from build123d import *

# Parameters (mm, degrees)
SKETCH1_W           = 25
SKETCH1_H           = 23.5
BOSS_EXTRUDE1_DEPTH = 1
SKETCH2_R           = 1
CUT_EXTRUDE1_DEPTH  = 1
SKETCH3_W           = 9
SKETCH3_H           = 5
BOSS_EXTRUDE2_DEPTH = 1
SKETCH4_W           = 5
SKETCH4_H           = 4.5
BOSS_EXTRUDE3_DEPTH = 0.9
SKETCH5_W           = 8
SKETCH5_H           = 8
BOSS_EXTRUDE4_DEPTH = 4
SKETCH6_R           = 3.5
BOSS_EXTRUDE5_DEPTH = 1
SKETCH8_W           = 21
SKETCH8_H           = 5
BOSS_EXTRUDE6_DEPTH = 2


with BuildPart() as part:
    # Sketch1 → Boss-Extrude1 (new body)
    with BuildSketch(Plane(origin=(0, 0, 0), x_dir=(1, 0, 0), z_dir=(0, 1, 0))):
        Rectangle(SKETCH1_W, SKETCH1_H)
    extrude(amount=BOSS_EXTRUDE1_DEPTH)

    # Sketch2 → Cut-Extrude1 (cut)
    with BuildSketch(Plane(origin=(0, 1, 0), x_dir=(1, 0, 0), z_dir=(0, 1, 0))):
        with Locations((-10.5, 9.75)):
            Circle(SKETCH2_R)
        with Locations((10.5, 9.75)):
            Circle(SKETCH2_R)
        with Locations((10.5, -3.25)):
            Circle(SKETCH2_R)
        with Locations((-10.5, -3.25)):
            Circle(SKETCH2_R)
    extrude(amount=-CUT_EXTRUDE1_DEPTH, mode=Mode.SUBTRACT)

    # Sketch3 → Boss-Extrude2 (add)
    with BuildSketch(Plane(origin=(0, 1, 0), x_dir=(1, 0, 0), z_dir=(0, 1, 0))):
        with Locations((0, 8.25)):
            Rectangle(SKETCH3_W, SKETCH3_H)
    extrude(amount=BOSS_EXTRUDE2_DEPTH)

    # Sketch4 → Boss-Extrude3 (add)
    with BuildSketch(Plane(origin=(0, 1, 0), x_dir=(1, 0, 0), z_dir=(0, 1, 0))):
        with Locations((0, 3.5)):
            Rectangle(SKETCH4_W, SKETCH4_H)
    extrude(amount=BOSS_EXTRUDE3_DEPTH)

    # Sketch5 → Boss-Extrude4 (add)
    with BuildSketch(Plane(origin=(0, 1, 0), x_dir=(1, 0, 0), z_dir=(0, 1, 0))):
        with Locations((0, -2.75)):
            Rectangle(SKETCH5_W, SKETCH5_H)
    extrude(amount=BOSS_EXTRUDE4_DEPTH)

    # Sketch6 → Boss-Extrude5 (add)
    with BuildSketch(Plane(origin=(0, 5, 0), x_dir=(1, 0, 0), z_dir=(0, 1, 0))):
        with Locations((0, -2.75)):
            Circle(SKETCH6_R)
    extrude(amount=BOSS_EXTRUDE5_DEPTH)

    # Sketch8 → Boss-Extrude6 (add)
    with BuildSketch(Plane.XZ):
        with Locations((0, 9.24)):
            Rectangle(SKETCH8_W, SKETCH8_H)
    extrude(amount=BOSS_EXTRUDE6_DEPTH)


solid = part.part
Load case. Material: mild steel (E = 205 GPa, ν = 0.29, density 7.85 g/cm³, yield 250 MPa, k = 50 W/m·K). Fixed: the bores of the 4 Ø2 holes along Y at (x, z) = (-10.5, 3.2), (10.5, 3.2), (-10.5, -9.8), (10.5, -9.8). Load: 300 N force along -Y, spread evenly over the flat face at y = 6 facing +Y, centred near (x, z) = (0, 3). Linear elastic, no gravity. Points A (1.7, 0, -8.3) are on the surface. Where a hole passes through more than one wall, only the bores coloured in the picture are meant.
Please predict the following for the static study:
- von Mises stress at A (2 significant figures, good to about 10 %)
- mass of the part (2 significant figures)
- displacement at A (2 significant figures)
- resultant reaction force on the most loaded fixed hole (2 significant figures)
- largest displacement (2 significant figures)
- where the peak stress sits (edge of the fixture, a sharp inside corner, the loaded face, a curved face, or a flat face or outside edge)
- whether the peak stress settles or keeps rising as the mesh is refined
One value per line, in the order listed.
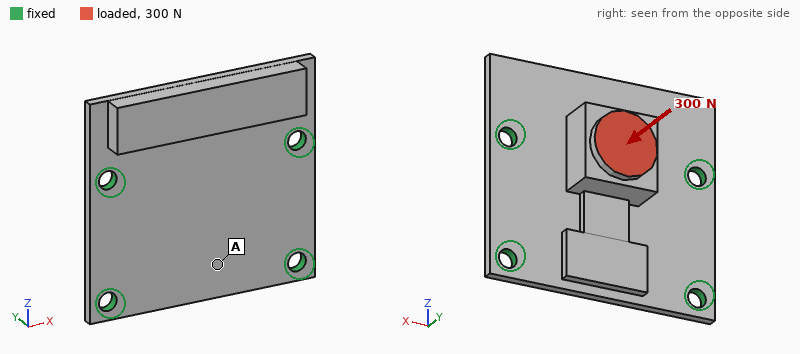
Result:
17 MPa
9.0 g
5.6 µm
140 N
15 µm
edge of the fixture
keeps rising
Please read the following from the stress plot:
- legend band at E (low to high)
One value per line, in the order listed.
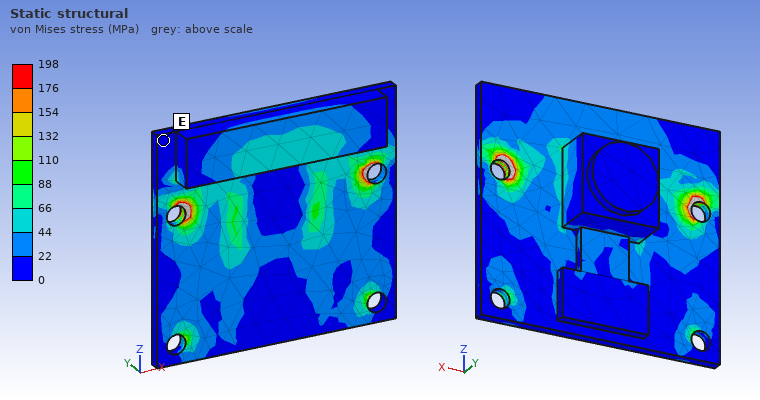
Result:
0 to 22 MPa
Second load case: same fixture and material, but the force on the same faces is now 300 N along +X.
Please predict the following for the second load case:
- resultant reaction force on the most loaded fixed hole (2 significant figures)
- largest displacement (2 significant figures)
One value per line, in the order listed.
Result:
140 N
7.6 µm
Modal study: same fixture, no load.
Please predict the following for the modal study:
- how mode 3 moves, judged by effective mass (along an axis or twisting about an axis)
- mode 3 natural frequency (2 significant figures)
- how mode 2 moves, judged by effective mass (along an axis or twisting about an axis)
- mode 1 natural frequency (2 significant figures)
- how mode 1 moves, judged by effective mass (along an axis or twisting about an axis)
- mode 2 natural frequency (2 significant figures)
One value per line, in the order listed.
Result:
twisting about Z
20 kHz
along Y
7800 Hz
along Y
12 kHz
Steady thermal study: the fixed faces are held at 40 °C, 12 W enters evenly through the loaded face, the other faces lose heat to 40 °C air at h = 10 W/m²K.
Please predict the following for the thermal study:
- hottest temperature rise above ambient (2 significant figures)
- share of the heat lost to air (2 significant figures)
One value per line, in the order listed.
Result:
79 K
3.9 %
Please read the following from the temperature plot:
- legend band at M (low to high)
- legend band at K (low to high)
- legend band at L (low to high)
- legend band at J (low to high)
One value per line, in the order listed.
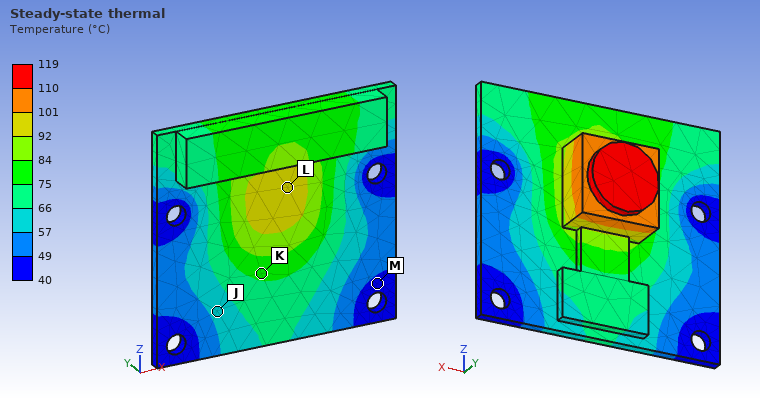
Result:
40 to 49 °C
75 to 84 °C
92 to 101 °C
57 to 66 °C
